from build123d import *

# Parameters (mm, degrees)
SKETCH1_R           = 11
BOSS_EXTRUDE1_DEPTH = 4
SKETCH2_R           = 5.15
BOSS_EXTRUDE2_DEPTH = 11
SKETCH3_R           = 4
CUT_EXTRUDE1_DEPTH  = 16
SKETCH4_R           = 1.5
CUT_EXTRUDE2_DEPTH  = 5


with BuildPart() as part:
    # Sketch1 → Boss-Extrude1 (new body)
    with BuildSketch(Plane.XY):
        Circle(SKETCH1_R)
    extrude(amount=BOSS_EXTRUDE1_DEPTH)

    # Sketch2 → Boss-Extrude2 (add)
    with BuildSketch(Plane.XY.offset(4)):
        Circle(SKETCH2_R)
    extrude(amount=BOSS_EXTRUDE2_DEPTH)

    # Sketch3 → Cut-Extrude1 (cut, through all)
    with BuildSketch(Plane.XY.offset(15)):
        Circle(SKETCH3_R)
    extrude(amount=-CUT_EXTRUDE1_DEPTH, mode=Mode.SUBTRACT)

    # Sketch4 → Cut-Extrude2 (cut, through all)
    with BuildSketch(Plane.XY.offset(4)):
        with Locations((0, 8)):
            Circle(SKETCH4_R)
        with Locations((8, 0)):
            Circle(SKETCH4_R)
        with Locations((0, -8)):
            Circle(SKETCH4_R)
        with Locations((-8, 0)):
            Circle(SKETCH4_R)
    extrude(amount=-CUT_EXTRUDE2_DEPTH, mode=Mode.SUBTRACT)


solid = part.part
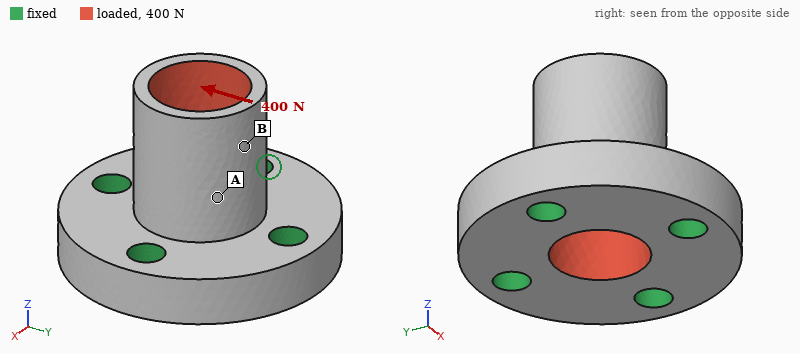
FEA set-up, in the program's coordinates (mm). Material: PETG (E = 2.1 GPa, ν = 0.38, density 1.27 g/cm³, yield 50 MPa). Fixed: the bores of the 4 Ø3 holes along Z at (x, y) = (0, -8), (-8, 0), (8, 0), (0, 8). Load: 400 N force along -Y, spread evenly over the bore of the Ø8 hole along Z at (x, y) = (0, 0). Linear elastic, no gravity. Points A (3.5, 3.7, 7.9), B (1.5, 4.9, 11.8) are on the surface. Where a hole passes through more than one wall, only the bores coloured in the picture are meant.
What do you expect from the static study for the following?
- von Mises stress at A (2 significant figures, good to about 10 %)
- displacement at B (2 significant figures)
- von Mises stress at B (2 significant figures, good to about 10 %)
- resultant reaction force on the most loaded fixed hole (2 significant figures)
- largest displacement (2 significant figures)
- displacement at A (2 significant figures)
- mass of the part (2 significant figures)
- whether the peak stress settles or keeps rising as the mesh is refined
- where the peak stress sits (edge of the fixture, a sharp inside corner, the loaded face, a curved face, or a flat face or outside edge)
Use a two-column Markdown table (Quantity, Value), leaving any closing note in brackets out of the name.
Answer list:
| Quantity | Value |
|---|---|
| von Mises stress at A | 13 MPa |
| displacement at B | 0.22 mm |
| von Mises stress at B | 5.2 MPa |
| resultant reaction force on the most loaded fixed hole | 190 N |
| largest displacement | 0.28 mm |
| displacement at A | 0.13 mm |
| mass of the part | 2.0 g |
| whether the peak stress settles or keeps rising as the mesh is refined | keeps rising |
| where the peak stress sits | a sharp inside corner |
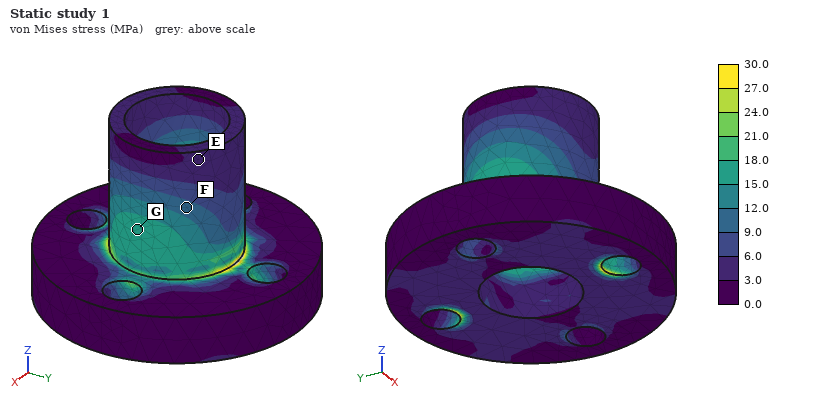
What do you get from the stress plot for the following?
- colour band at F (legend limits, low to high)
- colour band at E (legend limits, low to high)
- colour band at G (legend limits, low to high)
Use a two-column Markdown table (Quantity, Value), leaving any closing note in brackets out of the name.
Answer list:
| Quantity | Value |
|---|---|
| colour band at F | 9.0 to 12.0 MPa |
| colour band at E | 3.0 to 6.0 MPa |
| colour band at G | 15.0 to 18.0 MPa |
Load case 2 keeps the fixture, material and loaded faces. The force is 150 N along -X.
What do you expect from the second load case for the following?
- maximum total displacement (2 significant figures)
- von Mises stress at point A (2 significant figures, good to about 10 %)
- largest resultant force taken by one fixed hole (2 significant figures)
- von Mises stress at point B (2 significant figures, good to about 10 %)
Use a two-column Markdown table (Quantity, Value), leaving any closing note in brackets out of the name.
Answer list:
| Quantity | Value |
|---|---|
| maximum total displacement | 0.10 mm |
| von Mises stress at point A | 5.1 MPa |
| largest resultant force taken by one fixed hole | 72 N |
| von Mises stress at point B | 3.1 MPa |
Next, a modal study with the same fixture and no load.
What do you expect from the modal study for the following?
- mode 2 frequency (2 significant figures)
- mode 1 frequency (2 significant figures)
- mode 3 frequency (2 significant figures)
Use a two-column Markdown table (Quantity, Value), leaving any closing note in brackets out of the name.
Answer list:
| Quantity | Value |
|---|---|
| mode 2 frequency | 8900 Hz |
| mode 1 frequency | 8900 Hz |
| mode 3 frequency | 11 kHz |
